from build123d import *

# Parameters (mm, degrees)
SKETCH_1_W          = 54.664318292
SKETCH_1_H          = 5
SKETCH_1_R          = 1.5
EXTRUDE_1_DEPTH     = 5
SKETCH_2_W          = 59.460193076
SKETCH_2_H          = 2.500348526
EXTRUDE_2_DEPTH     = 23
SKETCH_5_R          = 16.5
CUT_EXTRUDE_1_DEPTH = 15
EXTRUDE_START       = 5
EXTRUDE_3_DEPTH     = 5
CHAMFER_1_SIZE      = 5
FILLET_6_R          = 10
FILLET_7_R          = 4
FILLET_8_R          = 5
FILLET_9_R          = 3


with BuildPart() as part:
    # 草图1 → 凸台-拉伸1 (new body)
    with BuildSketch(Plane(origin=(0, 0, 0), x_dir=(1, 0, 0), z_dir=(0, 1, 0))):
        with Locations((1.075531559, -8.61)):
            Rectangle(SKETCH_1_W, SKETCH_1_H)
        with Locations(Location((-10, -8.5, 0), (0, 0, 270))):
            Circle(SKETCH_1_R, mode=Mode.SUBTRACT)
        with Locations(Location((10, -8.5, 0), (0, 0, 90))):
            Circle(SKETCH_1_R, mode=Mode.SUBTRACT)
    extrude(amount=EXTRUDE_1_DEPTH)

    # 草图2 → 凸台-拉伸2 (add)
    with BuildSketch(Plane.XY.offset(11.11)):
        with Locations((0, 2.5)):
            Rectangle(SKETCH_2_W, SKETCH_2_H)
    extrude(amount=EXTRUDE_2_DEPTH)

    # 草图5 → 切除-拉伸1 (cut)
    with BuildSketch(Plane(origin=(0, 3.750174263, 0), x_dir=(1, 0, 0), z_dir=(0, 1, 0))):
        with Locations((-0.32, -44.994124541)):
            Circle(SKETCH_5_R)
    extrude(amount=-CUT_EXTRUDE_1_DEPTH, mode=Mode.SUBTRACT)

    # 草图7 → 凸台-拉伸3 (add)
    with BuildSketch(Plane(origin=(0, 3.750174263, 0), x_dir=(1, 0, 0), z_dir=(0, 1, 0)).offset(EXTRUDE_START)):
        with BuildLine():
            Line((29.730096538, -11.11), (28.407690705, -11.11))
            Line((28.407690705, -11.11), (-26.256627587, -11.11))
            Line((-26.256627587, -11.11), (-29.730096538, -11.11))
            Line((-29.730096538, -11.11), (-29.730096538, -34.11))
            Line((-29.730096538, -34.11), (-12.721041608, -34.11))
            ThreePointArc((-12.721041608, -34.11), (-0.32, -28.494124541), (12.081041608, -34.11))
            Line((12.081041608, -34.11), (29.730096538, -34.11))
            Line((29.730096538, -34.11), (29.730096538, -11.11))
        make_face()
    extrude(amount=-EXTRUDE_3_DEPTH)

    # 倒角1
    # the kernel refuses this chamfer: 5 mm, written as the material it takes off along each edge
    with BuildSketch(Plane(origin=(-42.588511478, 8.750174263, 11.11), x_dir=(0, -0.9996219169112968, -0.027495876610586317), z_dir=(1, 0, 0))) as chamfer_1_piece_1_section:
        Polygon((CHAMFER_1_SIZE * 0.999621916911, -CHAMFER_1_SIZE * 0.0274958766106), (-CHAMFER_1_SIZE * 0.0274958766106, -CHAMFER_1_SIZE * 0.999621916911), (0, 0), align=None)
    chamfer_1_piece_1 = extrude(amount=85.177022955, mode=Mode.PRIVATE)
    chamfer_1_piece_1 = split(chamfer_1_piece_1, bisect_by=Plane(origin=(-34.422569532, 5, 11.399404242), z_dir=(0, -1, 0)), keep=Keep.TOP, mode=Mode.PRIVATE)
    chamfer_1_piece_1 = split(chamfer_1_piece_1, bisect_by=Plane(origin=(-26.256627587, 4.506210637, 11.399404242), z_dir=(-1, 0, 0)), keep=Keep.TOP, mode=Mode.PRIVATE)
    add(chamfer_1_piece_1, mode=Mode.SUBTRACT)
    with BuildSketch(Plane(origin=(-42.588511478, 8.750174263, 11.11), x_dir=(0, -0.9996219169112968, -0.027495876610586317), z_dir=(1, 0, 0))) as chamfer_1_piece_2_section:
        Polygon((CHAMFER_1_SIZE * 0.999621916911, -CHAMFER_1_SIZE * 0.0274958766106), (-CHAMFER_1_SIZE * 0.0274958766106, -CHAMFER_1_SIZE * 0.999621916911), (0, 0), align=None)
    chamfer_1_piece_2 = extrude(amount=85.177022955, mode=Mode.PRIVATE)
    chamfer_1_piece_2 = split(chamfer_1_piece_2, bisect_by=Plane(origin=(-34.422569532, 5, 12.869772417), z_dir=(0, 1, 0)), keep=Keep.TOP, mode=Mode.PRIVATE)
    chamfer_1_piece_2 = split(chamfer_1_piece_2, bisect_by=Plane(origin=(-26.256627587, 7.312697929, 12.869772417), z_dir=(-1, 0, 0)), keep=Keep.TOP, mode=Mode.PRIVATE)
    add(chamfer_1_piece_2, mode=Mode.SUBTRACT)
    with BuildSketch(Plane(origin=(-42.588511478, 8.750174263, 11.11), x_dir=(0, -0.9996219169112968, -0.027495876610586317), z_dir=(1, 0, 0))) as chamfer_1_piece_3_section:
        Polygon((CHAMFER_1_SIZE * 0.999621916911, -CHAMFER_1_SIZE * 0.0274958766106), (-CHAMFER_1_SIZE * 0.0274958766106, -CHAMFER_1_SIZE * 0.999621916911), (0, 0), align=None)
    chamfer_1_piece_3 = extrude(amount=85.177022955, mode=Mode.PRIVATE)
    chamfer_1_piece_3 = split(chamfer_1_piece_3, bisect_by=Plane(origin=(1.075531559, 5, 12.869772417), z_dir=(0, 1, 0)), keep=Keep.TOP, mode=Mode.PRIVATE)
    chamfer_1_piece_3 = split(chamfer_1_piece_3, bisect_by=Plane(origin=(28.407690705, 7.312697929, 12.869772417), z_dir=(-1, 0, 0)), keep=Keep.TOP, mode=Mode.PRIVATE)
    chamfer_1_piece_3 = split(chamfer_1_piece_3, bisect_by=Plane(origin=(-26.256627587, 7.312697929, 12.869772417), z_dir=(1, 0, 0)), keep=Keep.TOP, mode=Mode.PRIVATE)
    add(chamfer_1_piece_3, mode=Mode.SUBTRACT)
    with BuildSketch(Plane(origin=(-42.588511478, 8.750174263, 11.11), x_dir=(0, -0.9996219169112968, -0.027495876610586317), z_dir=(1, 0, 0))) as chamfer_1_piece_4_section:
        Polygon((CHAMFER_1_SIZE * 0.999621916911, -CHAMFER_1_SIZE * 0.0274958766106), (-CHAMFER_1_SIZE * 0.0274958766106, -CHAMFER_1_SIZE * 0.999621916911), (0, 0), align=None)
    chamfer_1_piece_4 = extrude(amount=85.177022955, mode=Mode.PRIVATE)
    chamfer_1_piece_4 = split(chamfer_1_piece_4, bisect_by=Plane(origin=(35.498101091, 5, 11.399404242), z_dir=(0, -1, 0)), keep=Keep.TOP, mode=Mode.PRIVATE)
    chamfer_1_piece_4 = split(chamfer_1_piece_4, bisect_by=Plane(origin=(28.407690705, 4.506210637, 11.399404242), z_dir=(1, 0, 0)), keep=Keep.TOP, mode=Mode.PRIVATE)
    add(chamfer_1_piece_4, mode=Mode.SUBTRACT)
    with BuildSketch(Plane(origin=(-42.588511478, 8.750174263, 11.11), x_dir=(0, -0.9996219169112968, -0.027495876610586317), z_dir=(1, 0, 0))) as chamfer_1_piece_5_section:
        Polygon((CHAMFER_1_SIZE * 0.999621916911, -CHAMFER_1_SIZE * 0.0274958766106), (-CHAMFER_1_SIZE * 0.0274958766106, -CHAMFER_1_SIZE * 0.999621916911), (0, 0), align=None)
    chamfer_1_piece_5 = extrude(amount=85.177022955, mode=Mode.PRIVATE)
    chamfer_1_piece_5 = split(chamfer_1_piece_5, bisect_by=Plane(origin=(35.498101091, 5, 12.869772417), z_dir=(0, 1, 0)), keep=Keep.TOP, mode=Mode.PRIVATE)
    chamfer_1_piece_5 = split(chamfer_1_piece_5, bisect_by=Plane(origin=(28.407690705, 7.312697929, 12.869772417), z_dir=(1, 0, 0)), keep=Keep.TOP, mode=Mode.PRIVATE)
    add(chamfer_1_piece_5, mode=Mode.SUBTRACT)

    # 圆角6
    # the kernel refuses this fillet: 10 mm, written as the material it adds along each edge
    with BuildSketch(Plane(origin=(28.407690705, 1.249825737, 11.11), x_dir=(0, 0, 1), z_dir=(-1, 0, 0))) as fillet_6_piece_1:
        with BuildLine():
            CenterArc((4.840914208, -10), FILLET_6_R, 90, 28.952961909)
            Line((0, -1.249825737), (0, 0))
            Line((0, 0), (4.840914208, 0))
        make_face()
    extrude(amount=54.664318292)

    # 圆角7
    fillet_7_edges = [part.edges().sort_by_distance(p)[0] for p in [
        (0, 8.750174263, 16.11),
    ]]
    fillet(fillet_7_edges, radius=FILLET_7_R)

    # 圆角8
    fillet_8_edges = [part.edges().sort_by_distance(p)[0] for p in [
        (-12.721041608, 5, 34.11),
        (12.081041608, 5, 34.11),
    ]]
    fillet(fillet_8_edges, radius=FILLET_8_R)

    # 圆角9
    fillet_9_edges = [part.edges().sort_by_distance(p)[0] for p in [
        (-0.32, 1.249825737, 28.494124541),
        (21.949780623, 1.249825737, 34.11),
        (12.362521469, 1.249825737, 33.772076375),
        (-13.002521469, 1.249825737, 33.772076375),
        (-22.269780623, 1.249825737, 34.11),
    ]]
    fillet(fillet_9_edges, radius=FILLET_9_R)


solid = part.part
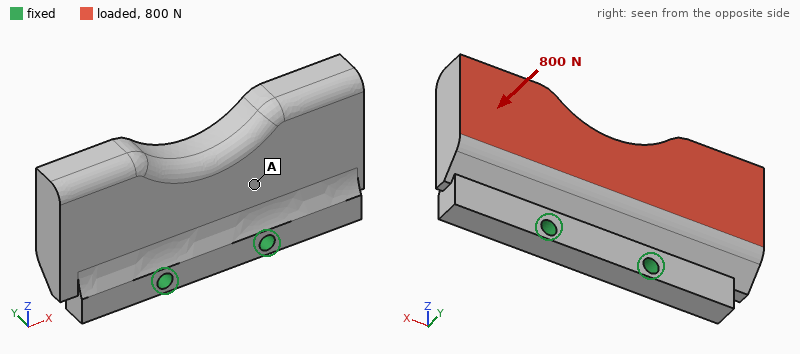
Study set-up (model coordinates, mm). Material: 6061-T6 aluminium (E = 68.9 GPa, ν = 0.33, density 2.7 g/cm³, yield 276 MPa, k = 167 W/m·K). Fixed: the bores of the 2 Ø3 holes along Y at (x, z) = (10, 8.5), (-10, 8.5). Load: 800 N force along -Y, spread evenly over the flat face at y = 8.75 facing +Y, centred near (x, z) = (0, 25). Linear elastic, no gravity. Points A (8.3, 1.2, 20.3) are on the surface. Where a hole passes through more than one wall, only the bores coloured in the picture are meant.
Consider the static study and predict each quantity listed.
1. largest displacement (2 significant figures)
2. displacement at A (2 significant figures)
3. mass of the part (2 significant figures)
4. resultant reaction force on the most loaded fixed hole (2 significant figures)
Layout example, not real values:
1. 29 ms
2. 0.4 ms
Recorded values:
1. 0.12 mm
2. 0.041 mm
3. 27 g
4. 400 N
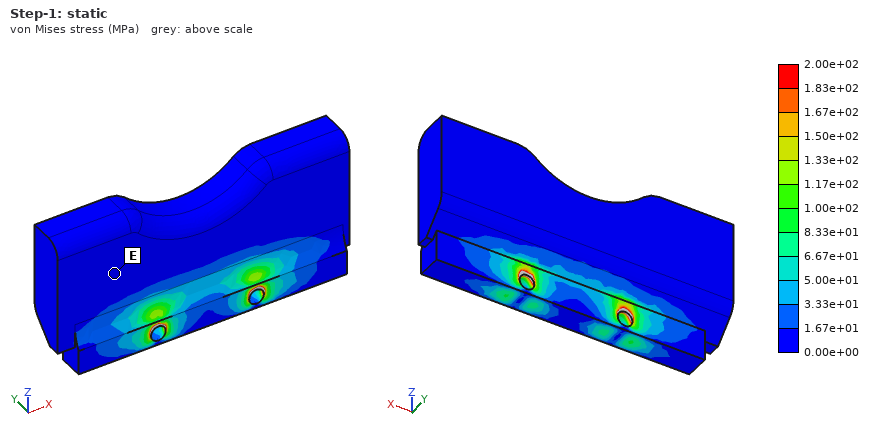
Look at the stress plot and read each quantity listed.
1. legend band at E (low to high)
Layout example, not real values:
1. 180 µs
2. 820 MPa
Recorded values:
1. 0.00e+00 to 1.67e+01 MPa
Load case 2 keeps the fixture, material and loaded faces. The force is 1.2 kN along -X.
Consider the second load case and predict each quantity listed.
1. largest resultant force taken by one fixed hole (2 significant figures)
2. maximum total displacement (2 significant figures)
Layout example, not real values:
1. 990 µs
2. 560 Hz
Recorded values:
1. 1.1 kN
2. 26 µm
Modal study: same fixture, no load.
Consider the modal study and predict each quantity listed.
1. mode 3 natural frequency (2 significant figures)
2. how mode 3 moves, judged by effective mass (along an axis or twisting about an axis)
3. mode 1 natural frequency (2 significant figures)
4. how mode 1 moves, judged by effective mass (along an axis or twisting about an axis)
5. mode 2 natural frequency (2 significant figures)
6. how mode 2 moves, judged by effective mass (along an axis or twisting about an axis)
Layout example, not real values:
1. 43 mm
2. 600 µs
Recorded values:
1. 10 kHz
2. along X
3. 3900 Hz
4. along Y
5. 5100 Hz
6. twisting about Z
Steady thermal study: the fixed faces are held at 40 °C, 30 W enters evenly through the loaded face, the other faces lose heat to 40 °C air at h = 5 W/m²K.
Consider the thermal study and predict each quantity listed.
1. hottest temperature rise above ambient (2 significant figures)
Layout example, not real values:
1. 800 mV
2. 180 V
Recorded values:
1. 15 K
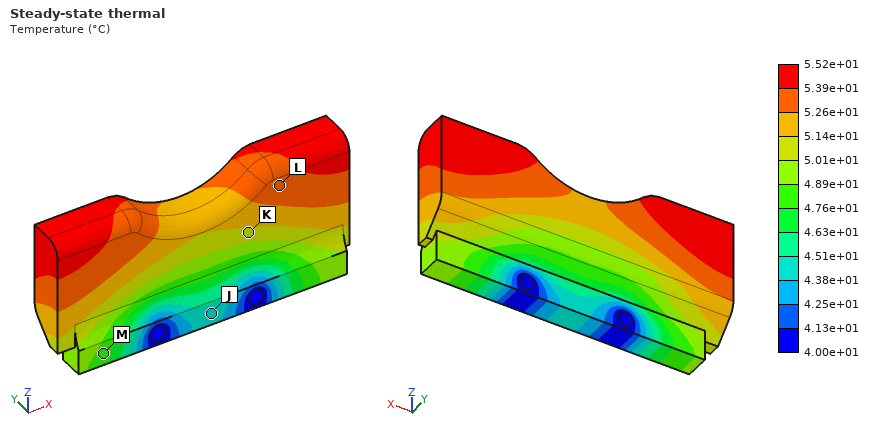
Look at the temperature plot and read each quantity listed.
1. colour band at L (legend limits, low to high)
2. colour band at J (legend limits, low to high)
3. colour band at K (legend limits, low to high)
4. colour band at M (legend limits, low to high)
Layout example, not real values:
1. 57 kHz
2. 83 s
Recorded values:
1. 5.26e+01 to 5.39e+01 °C
2. 4.38e+01 to 4.51e+01 °C
3. 5.01e+01 to 5.14e+01 °C
4. 4.76e+01 to 4.89e+01 °C
